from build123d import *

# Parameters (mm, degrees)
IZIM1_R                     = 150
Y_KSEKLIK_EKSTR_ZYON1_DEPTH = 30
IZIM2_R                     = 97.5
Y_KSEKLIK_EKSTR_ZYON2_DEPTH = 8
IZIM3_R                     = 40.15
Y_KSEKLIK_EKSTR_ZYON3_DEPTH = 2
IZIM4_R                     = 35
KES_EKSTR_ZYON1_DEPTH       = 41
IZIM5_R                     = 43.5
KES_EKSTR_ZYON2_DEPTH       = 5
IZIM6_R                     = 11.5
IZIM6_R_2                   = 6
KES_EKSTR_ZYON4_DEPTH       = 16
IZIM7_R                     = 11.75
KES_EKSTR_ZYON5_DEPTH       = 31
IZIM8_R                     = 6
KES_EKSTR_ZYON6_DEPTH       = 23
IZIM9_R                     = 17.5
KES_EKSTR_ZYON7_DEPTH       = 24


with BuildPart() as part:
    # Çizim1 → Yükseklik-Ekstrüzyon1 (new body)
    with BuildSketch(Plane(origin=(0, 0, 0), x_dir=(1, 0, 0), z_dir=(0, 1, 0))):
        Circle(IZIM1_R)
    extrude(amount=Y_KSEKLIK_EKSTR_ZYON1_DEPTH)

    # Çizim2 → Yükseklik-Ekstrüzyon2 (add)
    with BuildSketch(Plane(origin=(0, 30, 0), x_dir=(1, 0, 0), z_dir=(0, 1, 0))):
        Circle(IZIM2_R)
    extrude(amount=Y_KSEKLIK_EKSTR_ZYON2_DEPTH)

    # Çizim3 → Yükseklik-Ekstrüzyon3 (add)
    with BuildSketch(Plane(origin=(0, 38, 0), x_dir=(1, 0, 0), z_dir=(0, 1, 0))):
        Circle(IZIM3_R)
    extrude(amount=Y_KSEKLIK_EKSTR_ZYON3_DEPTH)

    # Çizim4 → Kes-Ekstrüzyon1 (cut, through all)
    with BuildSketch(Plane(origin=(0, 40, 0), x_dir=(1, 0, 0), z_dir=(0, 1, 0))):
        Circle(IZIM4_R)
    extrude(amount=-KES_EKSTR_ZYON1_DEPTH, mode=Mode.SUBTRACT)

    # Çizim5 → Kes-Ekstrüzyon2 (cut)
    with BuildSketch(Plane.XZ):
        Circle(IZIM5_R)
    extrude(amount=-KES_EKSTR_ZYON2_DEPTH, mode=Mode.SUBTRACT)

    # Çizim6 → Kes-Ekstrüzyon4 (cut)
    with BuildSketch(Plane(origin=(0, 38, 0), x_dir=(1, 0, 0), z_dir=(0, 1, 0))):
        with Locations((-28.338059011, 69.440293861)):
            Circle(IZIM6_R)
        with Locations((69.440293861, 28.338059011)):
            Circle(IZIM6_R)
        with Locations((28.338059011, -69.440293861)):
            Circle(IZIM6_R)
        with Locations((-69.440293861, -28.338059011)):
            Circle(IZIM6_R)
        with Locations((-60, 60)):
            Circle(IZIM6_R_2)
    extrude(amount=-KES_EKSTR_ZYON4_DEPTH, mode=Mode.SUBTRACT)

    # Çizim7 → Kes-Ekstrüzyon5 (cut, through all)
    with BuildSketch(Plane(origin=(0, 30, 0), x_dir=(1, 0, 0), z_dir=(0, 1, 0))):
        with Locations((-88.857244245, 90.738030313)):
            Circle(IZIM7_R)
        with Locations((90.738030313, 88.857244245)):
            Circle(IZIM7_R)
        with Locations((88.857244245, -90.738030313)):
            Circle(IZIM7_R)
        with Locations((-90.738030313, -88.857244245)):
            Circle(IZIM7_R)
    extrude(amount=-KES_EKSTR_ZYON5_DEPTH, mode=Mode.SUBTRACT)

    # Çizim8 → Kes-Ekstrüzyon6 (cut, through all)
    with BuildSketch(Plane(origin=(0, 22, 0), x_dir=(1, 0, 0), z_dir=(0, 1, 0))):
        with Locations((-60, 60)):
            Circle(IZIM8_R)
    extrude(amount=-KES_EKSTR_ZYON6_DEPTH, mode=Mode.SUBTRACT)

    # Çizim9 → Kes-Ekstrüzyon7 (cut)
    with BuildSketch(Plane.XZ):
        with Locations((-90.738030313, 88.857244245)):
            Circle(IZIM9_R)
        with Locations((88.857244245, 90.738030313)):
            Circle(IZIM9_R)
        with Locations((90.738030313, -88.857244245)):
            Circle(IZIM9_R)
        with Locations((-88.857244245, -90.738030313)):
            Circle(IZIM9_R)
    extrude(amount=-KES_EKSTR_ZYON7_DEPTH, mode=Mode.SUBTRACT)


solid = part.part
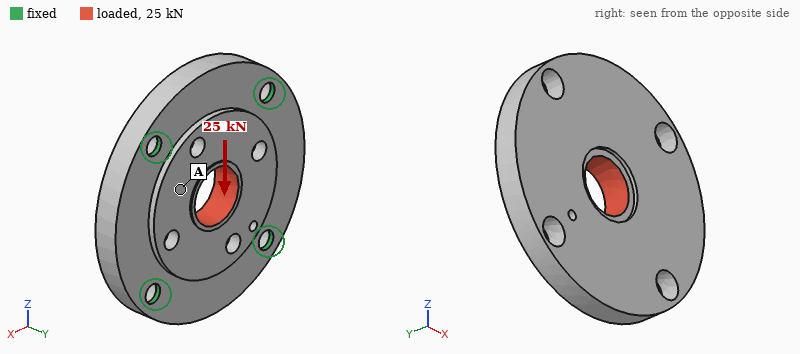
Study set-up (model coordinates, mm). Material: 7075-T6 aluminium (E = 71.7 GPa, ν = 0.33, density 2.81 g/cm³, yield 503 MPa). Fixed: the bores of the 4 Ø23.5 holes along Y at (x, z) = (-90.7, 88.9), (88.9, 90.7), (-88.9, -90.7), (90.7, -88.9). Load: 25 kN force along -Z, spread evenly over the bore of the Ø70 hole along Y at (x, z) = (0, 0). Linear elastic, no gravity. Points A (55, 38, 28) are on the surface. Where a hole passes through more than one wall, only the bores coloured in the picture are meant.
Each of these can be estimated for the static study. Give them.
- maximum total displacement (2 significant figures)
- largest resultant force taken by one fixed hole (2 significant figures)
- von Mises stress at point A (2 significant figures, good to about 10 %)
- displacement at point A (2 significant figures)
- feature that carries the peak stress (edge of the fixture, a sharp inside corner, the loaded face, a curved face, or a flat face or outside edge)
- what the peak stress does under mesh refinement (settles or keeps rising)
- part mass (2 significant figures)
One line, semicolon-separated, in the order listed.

10 µm; 6.4 kN; 2.8 MPa; 7.0 µm; edge of the fixture; keeps rising; 5.8 kg
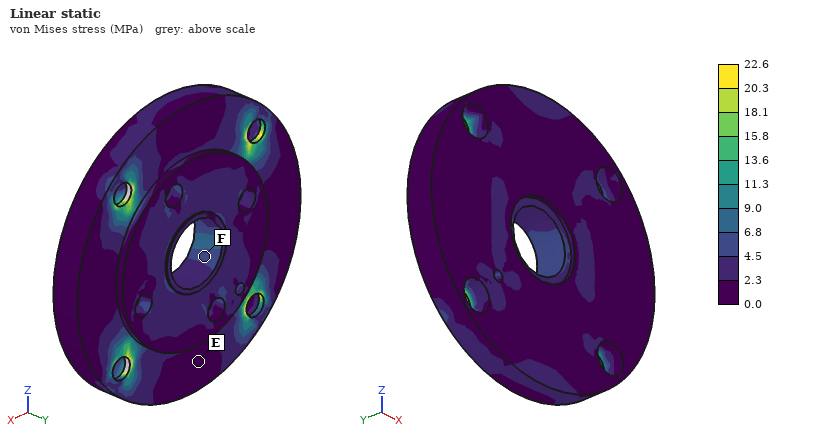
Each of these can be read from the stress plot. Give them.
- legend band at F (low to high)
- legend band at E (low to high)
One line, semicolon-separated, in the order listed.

4.5 to 6.8 MPa; 0.0 to 2.3 MPa
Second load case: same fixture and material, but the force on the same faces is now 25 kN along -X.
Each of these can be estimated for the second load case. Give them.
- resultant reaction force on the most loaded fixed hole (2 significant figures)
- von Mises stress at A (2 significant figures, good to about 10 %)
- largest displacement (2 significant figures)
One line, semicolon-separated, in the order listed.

6.4 kN; 3.3 MPa; 10 µm
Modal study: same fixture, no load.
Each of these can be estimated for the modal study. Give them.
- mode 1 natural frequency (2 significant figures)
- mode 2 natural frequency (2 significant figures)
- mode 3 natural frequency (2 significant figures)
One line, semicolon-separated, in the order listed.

2400 Hz; 2400 Hz; 2700 Hz
